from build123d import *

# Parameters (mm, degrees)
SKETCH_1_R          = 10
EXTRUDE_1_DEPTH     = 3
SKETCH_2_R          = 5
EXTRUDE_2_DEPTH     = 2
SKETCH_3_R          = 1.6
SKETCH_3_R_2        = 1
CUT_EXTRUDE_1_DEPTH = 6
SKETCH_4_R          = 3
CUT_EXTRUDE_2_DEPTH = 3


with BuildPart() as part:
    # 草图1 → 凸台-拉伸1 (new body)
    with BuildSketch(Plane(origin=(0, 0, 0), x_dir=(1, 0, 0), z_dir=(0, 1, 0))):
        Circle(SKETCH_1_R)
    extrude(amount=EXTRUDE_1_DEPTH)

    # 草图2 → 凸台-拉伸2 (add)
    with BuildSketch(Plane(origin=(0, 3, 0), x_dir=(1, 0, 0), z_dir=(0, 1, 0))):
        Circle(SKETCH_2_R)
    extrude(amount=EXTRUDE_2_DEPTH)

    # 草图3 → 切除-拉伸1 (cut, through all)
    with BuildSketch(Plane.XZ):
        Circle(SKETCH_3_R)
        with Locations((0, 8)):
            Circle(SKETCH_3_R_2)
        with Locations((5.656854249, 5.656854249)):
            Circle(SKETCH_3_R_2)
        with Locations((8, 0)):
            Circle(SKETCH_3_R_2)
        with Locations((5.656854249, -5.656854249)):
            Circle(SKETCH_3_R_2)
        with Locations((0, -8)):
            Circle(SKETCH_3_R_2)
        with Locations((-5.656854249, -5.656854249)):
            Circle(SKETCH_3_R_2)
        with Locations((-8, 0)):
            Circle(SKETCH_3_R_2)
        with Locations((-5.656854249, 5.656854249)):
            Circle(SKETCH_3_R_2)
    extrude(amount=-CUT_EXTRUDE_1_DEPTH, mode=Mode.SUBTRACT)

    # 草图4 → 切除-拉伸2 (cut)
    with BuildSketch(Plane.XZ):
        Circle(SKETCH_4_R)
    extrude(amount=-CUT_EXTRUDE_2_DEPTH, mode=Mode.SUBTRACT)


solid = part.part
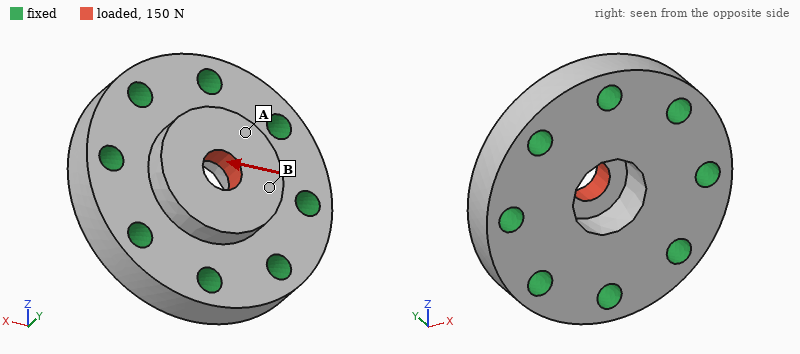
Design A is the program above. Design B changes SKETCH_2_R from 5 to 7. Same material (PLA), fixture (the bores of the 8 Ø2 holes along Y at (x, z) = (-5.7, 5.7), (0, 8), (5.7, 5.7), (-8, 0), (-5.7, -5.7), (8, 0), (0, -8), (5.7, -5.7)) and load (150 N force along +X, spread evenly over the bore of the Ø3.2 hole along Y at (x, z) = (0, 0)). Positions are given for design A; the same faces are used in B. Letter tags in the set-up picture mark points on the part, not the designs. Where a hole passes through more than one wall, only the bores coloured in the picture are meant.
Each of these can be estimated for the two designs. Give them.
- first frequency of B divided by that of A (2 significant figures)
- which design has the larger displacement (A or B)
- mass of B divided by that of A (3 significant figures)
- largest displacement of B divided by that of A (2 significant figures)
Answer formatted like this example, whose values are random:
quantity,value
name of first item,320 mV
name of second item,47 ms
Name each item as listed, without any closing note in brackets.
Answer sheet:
quantity,value
first frequency of B divided by that of A,1.1
which design has the larger displacement,A
mass of B divided by that of A,1.16
largest displacement of B divided by that of A,0.72
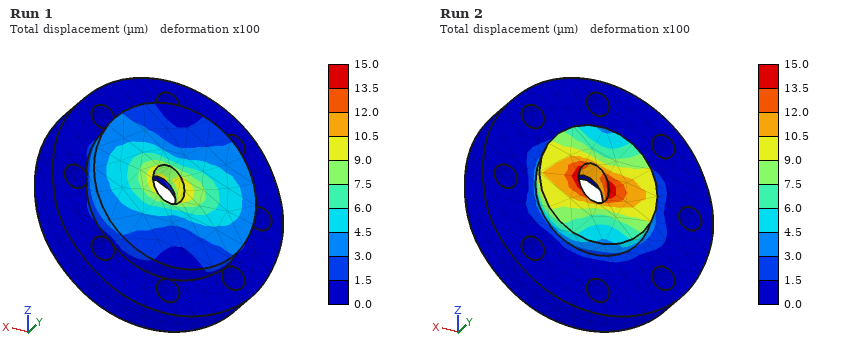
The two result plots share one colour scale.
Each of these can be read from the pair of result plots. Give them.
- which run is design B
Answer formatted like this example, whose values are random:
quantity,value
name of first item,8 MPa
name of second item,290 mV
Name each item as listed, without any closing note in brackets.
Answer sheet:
quantity,value
which run is design B,Run 1
